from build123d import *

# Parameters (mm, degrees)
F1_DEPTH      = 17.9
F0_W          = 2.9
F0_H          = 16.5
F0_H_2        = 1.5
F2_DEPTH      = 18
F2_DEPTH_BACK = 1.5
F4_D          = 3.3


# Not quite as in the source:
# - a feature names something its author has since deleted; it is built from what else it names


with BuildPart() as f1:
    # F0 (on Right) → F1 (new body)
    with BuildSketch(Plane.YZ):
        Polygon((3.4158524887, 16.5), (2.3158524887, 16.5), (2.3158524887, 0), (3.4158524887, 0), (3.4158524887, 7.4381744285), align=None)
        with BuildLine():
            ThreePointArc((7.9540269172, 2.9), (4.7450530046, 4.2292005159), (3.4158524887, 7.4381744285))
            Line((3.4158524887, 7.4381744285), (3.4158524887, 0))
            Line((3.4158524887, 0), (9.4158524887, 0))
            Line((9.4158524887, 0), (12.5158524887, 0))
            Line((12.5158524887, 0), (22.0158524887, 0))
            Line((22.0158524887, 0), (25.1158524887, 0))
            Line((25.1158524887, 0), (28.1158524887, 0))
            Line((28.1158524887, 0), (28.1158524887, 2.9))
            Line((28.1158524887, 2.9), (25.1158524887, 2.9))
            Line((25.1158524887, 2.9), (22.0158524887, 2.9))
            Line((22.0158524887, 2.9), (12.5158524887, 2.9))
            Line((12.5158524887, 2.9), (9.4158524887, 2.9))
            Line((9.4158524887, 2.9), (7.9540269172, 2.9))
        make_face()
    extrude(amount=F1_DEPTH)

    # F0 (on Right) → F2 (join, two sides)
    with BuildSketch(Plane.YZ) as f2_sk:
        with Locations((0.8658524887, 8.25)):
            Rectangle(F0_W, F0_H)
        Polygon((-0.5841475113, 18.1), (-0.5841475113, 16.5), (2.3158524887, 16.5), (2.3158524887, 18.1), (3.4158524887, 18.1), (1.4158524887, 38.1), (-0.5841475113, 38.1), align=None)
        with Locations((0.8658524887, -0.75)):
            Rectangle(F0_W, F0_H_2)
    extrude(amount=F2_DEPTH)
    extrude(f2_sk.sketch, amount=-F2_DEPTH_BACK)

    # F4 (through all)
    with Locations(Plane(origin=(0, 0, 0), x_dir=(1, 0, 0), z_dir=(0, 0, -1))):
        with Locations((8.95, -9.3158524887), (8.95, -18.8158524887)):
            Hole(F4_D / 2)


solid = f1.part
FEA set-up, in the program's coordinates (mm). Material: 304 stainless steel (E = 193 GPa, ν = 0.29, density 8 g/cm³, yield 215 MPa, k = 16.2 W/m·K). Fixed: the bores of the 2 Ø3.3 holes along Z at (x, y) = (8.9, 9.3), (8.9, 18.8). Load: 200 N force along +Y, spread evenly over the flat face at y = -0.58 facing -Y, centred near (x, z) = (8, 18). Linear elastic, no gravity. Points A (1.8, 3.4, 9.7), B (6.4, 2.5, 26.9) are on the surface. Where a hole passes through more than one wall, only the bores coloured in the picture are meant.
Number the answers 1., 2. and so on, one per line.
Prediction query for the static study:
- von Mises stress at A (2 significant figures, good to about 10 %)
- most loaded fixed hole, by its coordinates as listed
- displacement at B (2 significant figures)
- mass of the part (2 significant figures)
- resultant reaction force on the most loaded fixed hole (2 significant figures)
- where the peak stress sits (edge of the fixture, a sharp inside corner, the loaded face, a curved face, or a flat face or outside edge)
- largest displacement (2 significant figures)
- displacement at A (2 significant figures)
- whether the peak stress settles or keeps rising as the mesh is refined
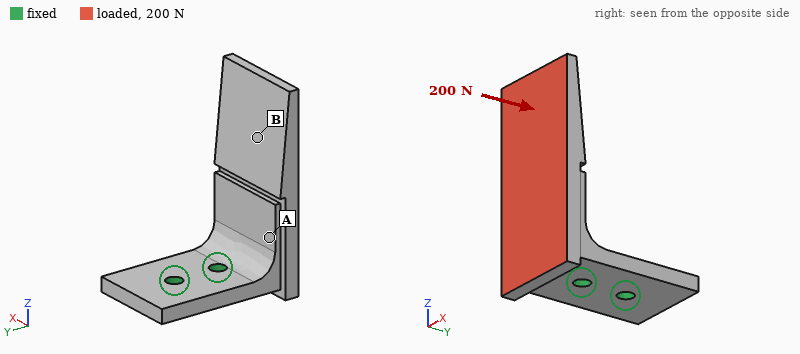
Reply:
1. 41 MPa
2. (8.9, 9.3)
3. 0.081 mm
4. 31 g
5. 210 N
6. edge of the fixture
7. 0.13 mm
8. 0.020 mm
9. keeps rising
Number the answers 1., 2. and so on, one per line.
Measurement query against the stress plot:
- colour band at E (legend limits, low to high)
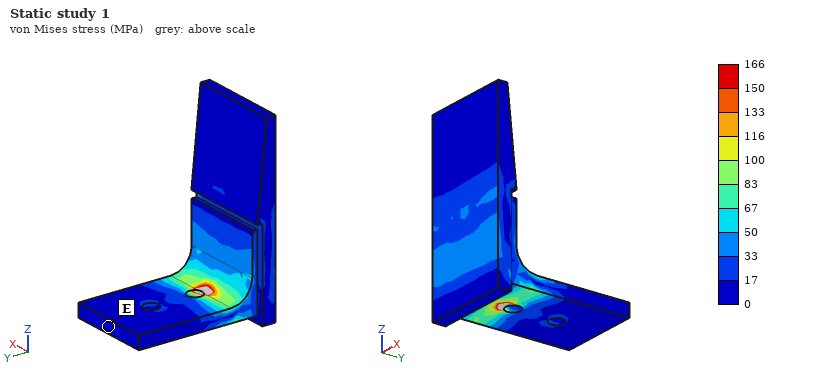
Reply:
1. 0 to 17 MPa
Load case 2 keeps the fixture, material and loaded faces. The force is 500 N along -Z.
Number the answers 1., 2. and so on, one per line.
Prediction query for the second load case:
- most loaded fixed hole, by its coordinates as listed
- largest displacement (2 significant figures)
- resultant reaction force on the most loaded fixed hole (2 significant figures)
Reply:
1. (8.9, 9.3)
2. 0.11 mm
3. 640 N
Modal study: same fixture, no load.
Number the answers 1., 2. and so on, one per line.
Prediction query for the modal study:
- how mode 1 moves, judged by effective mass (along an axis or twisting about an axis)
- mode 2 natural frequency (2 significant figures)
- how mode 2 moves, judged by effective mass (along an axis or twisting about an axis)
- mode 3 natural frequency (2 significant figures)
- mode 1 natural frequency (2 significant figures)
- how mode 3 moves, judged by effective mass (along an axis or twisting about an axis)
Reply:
1. along Y
2. 2900 Hz
3. along X
4. 8500 Hz
5. 1900 Hz
6. along Z
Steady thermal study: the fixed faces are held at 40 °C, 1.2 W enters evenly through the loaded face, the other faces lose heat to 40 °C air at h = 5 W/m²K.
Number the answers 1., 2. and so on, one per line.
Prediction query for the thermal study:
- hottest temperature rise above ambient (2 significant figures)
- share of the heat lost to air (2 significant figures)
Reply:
1. 24 K
2. 8.9 %
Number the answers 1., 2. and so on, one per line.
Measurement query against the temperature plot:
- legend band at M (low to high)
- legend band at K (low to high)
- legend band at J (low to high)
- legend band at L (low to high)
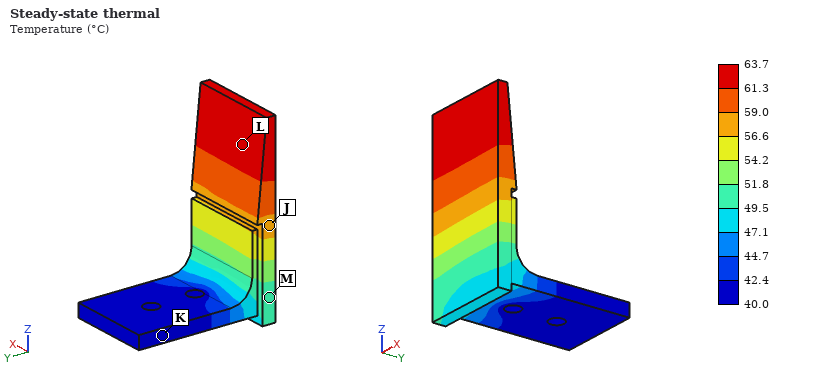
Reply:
1. 49.5 to 51.8 °C
2. 40.0 to 42.4 °C
3. 56.6 to 59.0 °C
4. 61.3 to 63.7 °C
